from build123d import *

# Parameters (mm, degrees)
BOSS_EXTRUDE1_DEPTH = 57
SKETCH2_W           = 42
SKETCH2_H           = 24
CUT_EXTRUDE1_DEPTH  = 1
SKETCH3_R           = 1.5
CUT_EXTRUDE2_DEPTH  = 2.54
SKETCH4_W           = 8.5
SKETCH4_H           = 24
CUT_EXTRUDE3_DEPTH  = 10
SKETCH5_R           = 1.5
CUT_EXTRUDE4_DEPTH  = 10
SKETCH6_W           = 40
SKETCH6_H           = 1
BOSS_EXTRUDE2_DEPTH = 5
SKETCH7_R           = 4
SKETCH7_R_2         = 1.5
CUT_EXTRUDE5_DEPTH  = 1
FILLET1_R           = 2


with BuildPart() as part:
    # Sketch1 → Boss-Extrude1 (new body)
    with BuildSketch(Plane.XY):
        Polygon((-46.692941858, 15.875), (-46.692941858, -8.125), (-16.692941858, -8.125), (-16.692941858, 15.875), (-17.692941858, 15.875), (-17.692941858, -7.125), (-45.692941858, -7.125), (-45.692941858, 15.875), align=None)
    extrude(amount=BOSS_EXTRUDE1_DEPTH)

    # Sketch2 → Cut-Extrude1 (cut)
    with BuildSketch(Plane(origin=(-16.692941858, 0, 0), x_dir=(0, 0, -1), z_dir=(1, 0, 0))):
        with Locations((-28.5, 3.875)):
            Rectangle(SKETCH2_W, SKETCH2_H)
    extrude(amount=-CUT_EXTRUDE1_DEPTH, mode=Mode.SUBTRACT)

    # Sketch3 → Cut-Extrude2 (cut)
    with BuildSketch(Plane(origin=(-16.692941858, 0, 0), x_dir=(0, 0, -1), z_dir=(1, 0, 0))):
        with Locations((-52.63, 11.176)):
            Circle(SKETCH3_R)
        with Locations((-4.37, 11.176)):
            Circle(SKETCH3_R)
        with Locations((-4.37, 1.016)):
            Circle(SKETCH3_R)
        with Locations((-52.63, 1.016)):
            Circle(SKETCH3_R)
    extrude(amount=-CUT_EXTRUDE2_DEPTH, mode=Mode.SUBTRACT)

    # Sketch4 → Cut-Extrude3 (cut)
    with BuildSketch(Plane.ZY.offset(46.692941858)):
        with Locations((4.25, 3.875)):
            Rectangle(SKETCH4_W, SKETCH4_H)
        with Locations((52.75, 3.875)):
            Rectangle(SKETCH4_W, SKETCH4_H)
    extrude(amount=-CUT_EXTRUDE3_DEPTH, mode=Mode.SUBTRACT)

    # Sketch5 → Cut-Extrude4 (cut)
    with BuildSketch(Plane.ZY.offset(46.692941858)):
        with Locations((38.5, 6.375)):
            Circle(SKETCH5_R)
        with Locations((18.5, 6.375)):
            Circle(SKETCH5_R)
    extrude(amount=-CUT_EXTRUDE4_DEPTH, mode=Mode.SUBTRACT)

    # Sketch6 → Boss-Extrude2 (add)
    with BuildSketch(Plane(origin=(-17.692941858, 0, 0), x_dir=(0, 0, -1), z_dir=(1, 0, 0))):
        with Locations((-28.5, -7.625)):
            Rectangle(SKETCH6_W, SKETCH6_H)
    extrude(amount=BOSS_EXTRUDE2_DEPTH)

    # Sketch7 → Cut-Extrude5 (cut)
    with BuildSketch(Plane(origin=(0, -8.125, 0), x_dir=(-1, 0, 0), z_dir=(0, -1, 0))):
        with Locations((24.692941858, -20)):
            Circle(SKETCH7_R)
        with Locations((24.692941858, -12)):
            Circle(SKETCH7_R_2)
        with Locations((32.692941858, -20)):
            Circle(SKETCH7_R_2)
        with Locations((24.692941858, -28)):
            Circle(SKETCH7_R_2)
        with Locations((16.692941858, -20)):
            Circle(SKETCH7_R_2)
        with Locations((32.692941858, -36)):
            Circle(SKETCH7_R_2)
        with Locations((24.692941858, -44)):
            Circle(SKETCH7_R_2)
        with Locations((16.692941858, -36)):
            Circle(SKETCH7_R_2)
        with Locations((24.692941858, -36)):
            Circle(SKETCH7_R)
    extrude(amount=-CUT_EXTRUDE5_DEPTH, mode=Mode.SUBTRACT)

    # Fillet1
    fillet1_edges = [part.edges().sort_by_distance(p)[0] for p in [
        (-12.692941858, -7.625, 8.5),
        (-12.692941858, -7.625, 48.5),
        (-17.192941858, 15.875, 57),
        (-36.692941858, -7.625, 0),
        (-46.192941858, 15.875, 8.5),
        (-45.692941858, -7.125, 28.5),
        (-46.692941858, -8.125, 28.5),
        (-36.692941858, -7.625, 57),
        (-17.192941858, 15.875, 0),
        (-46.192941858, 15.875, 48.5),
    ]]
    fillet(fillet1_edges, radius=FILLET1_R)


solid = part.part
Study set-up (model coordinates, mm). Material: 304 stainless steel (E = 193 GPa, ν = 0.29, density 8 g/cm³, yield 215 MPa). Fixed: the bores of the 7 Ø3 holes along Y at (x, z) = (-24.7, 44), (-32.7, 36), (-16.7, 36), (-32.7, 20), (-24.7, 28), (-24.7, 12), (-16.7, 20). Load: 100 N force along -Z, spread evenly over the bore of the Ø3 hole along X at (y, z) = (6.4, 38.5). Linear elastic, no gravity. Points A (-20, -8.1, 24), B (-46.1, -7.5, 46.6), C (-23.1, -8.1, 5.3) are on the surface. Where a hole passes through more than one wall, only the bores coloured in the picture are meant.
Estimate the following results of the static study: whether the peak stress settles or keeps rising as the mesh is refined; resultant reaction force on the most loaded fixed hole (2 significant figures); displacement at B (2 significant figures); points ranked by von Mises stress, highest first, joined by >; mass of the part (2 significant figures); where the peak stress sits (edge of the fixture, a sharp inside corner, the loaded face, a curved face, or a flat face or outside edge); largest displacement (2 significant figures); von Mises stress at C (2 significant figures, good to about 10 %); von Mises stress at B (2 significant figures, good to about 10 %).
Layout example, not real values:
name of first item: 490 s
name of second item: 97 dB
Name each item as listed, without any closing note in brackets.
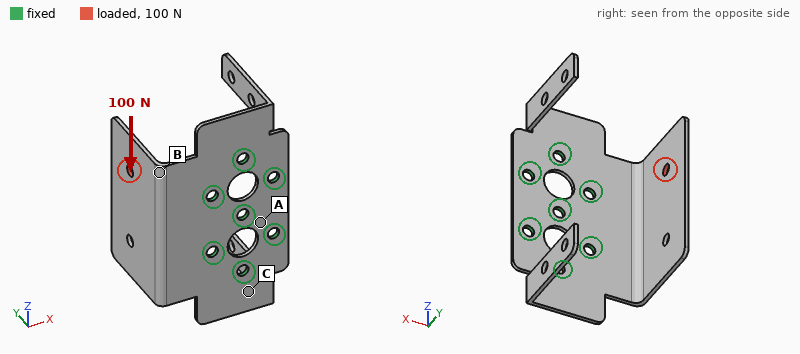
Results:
whether the peak stress settles or keeps rising as the mesh is refined: keeps rising
resultant reaction force on the most loaded fixed hole: 79 N
displacement at B: 0.11 mm
points ranked by von Mises stress, highest first, joined by >: B > C > A
mass of the part: 22 g
where the peak stress sits: edge of the fixture
largest displacement: 0.19 mm
von Mises stress at C: 23 MPa
von Mises stress at B: 42 MPa
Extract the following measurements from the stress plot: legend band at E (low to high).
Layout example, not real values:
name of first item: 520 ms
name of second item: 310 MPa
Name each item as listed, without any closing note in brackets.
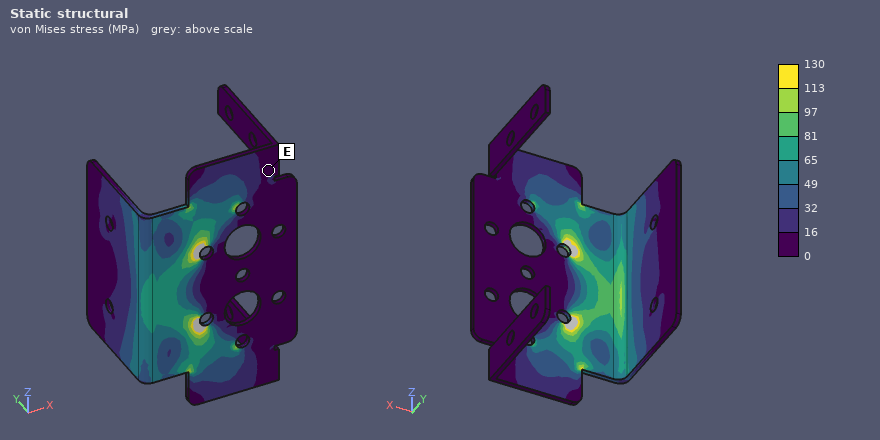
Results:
legend band at E: 0 to 16 MPa
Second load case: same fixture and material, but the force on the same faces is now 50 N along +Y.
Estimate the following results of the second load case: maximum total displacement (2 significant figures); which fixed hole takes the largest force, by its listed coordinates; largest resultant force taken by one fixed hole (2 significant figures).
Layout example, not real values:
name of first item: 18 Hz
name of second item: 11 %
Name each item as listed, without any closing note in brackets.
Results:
maximum total displacement: 0.21 mm
which fixed hole takes the largest force, by its listed coordinates: (-32.7, 36)
largest resultant force taken by one fixed hole: 57 N
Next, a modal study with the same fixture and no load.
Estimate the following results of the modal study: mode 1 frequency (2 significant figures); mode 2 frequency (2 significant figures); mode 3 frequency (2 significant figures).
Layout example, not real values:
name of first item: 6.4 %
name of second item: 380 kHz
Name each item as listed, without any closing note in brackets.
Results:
mode 1 frequency: 810 Hz
mode 2 frequency: 1100 Hz
mode 3 frequency: 1100 Hz
